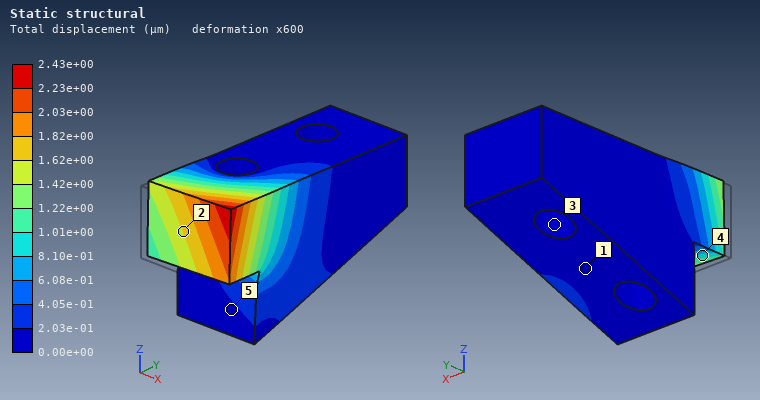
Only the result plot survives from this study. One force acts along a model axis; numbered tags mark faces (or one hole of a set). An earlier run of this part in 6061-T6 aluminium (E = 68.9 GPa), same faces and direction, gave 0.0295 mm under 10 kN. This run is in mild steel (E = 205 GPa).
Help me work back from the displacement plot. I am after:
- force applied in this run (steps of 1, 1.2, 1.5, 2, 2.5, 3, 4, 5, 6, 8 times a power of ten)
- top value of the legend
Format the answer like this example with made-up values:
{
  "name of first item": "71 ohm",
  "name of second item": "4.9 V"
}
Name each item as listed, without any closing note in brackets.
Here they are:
{
  "force applied in this run": "2.5 kN",
  "top value of the legend": "2.43e+00 µm"
}
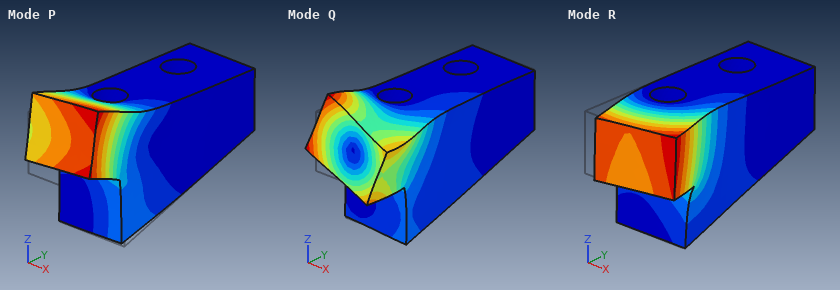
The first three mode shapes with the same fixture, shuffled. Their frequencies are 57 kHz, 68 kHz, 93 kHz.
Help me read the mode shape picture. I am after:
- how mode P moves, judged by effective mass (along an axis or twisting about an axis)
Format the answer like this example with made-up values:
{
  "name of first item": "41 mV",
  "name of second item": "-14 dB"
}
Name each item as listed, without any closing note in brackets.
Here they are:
{
  "how mode P moves, judged by effective mass": "along Z"
}
